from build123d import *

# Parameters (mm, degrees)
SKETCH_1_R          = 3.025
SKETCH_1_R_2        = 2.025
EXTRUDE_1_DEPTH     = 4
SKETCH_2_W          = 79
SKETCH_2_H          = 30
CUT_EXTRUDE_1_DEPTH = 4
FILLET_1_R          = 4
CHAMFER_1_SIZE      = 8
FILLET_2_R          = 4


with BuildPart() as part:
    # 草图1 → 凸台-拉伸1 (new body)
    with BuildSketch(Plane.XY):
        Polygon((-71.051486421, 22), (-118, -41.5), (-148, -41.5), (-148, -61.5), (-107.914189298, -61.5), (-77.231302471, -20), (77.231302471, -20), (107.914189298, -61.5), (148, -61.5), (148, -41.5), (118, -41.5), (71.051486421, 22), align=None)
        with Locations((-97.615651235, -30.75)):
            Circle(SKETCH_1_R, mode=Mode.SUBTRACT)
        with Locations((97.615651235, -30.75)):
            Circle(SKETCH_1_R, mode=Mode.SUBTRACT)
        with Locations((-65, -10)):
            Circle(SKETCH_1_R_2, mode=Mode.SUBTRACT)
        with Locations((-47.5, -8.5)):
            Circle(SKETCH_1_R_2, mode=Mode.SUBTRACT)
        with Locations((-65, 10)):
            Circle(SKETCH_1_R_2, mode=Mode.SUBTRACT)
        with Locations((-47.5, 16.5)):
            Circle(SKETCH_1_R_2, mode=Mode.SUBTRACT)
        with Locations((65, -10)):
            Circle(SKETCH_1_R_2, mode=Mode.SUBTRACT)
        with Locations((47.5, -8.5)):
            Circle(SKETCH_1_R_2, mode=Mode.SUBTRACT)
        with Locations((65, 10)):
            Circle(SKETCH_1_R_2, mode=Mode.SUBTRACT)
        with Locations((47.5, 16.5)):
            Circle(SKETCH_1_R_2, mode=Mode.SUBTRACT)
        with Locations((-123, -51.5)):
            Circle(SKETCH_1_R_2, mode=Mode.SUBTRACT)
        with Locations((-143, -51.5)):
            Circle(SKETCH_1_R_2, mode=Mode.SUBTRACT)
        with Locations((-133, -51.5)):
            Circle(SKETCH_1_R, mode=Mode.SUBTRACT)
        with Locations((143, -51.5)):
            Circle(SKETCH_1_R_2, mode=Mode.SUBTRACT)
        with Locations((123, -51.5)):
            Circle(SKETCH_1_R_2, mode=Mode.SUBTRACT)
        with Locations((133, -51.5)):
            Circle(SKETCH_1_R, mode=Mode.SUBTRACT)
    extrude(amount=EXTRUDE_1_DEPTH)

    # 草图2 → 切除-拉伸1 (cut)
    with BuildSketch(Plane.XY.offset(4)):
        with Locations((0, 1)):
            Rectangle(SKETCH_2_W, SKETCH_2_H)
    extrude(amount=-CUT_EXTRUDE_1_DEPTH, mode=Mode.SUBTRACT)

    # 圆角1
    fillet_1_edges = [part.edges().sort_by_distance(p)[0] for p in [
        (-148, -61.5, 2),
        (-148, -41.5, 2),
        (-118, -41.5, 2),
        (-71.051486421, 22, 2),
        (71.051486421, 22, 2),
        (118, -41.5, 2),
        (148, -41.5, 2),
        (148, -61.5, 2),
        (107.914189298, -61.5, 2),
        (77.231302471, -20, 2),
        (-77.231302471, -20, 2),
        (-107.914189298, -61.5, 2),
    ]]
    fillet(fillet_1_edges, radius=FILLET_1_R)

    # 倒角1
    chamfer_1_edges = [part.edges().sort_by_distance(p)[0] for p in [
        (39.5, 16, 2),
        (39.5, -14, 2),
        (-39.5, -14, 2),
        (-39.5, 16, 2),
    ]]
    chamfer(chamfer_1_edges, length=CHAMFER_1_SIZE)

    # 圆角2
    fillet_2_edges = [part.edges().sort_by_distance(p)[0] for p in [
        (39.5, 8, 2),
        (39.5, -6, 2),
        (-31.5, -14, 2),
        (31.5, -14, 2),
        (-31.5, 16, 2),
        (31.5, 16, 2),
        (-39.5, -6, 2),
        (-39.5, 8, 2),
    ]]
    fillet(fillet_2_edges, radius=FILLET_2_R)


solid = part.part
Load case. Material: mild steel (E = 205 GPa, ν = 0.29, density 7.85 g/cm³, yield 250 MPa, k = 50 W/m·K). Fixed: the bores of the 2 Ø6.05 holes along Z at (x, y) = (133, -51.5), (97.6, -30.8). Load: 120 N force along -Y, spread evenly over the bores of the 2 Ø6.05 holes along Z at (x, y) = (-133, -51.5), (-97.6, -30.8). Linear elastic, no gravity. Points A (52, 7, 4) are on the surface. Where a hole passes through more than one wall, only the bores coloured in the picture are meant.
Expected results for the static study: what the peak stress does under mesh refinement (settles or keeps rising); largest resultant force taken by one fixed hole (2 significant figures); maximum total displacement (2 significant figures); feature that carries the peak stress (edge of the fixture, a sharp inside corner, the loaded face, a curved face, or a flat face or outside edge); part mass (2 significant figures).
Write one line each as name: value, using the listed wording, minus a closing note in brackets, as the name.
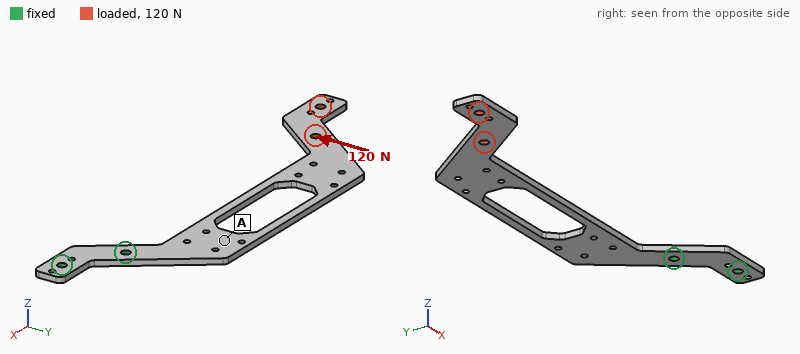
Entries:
what the peak stress does under mesh refinement: keeps rising
largest resultant force taken by one fixed hole: 470 N
maximum total displacement: 0.65 mm
feature that carries the peak stress: edge of the fixture
part mass: 240 g
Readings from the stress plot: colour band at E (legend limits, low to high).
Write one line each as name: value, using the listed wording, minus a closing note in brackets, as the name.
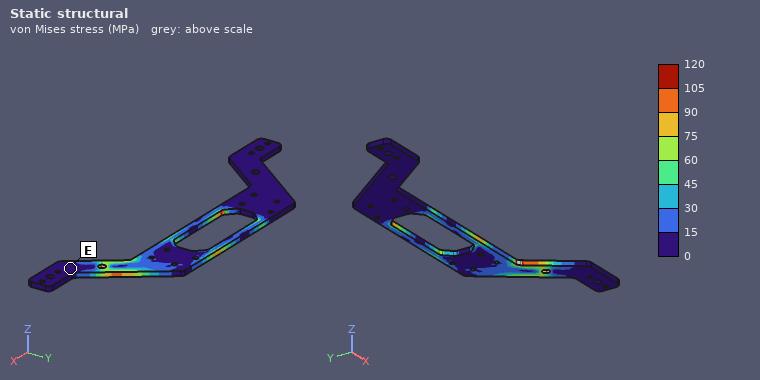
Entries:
colour band at E: 0 to 15 MPa
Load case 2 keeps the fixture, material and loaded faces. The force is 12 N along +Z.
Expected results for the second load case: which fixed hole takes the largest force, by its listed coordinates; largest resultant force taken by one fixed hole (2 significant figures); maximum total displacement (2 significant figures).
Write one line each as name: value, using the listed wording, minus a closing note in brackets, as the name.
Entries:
which fixed hole takes the largest force, by its listed coordinates: (97.6, -30.8)
largest resultant force taken by one fixed hole: 12 N
maximum total displacement: 2.5 mm
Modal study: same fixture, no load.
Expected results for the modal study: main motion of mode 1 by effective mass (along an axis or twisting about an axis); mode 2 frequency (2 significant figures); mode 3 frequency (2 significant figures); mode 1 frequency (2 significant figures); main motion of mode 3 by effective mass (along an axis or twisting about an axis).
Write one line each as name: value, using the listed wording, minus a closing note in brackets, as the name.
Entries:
main motion of mode 1 by effective mass: along Z
mode 2 frequency: 210 Hz
mode 3 frequency: 250 Hz
mode 1 frequency: 46 Hz
main motion of mode 3 by effective mass: along Y
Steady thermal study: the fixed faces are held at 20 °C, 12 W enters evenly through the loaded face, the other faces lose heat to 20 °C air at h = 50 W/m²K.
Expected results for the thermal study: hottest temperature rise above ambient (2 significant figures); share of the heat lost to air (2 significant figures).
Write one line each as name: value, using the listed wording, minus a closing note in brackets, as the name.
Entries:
hottest temperature rise above ambient: 61 K
share of the heat lost to air: 100 %
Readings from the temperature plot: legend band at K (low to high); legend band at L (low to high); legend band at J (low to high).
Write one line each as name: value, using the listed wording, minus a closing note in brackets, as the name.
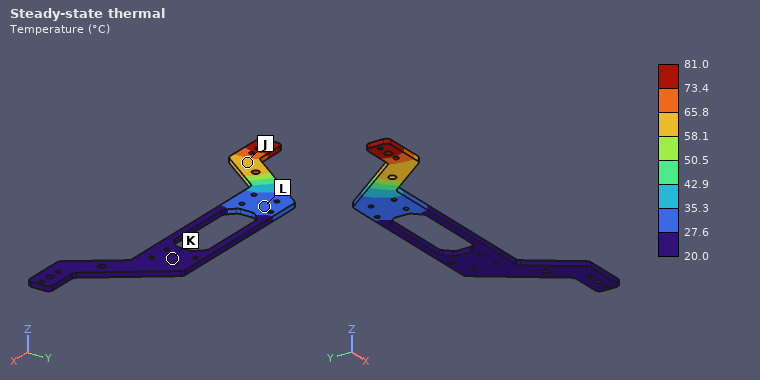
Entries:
legend band at K: 20.0 to 27.6 °C
legend band at L: 27.6 to 35.3 °C
legend band at J: 58.1 to 65.8 °C
